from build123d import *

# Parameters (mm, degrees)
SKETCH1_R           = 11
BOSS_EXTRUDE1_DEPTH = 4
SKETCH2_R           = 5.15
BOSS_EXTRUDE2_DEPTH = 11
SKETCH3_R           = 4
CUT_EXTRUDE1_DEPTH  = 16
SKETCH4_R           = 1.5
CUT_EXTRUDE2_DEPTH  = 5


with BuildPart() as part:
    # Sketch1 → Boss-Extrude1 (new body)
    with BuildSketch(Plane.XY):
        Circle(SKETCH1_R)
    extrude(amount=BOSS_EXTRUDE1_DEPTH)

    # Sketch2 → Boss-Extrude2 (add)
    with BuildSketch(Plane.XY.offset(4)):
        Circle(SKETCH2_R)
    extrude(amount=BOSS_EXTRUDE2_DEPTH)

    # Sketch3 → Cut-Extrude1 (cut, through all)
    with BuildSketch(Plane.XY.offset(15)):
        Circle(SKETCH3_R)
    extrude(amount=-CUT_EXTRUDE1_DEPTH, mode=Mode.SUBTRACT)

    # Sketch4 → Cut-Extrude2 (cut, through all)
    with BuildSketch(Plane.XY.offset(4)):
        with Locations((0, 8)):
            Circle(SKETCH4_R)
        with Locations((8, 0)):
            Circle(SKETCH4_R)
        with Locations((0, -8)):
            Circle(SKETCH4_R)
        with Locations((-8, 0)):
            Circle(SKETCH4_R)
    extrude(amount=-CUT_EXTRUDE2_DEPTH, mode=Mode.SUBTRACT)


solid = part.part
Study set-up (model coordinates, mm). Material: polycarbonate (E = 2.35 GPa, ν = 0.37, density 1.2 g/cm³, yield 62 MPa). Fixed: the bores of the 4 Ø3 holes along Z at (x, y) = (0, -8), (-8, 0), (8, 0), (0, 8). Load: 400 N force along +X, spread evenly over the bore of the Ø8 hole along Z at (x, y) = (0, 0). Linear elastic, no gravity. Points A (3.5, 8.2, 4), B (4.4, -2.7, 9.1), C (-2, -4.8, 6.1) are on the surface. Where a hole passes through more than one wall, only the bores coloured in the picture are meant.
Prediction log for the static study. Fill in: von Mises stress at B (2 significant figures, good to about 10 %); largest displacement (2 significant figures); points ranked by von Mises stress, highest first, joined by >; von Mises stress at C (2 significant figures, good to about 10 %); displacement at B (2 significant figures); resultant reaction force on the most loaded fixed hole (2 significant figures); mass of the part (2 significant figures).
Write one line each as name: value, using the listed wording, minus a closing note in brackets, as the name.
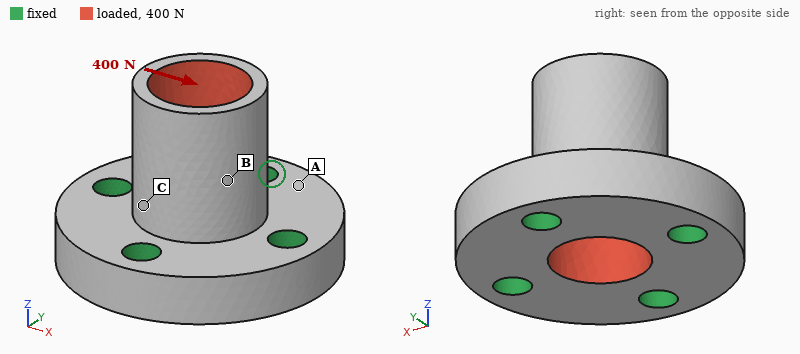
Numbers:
von Mises stress at B: 10 MPa
largest displacement: 0.25 mm
points ranked by von Mises stress, highest first, joined by >: C > B > A
von Mises stress at C: 17 MPa
displacement at B: 0.15 mm
resultant reaction force on the most loaded fixed hole: 190 N
mass of the part: 1.9 g
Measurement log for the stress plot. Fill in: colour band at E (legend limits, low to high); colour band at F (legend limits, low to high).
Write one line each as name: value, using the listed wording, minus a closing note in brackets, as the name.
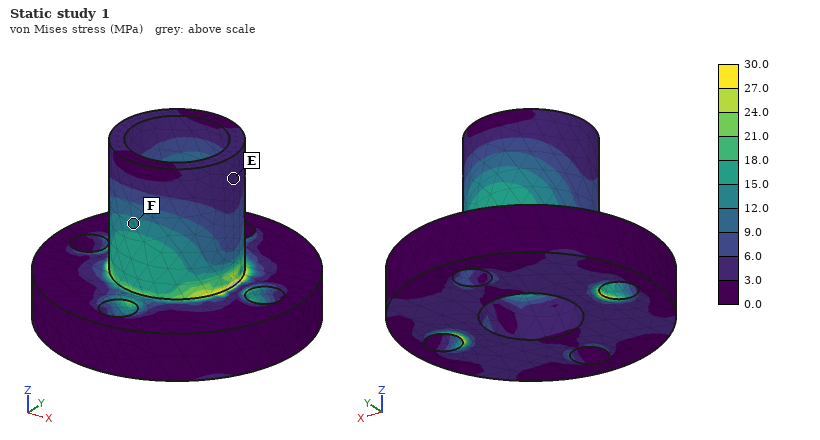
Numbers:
colour band at E: 3.0 to 6.0 MPa
colour band at F: 12.0 to 15.0 MPa
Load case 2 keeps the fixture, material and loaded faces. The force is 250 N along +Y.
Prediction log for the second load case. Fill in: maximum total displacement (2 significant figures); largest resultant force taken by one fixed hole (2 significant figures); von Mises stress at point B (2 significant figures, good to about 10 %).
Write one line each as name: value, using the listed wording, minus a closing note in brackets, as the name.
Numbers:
maximum total displacement: 0.16 mm
largest resultant force taken by one fixed hole: 120 N
von Mises stress at point B: 8.4 MPa
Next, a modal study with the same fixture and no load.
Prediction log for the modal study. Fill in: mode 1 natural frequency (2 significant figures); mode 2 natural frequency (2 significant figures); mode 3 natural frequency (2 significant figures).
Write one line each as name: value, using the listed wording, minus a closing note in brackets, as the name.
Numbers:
mode 1 natural frequency: 9600 Hz
mode 2 natural frequency: 9700 Hz
mode 3 natural frequency: 11 kHz
